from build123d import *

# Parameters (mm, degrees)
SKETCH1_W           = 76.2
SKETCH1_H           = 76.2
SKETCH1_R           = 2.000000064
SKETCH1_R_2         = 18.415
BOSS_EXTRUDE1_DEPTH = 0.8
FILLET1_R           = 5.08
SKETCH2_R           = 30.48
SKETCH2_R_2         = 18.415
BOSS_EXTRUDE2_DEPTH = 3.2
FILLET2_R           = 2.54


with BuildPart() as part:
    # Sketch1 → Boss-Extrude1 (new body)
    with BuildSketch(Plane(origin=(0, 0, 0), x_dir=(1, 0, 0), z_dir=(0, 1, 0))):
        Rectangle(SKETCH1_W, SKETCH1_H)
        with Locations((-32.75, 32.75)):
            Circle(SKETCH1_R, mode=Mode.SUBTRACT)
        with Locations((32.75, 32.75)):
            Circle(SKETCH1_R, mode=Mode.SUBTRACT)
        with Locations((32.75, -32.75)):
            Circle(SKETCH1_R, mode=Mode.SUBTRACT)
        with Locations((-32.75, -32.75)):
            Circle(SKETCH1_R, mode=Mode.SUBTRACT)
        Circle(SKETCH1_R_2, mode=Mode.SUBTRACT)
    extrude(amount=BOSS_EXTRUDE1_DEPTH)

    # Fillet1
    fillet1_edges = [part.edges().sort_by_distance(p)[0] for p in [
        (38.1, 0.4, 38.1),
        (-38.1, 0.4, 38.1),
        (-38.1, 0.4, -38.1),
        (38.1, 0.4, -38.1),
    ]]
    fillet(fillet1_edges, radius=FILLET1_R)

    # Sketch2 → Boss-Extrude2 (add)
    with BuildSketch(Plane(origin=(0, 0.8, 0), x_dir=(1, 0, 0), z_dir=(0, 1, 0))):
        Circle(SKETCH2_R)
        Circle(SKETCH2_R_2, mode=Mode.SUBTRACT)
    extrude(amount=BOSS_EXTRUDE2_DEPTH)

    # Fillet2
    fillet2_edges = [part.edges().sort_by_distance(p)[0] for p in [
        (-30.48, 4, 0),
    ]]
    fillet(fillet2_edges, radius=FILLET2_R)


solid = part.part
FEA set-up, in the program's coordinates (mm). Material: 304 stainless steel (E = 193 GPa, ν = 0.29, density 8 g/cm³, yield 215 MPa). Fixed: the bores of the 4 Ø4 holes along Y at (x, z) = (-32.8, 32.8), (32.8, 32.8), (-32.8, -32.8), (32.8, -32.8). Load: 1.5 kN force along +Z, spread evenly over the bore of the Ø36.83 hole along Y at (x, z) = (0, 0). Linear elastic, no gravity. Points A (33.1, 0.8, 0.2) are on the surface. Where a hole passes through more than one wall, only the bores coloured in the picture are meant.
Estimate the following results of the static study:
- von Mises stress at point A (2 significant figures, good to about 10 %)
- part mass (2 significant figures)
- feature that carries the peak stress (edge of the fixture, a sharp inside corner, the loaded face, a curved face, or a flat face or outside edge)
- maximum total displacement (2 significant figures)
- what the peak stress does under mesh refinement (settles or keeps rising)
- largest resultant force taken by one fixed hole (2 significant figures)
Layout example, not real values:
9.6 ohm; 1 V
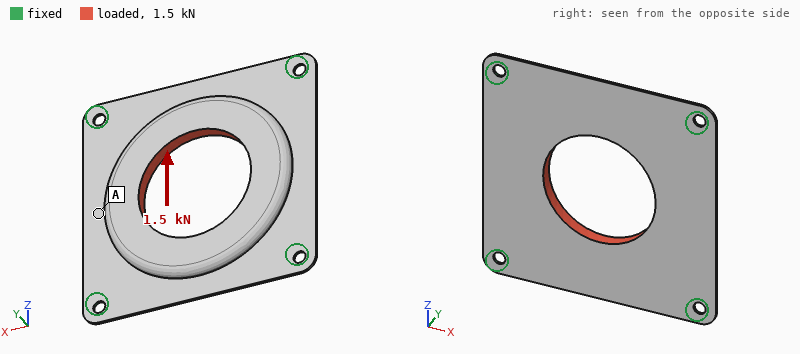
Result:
13 MPa; 75 g; edge of the fixture; 48 µm; keeps rising; 400 N
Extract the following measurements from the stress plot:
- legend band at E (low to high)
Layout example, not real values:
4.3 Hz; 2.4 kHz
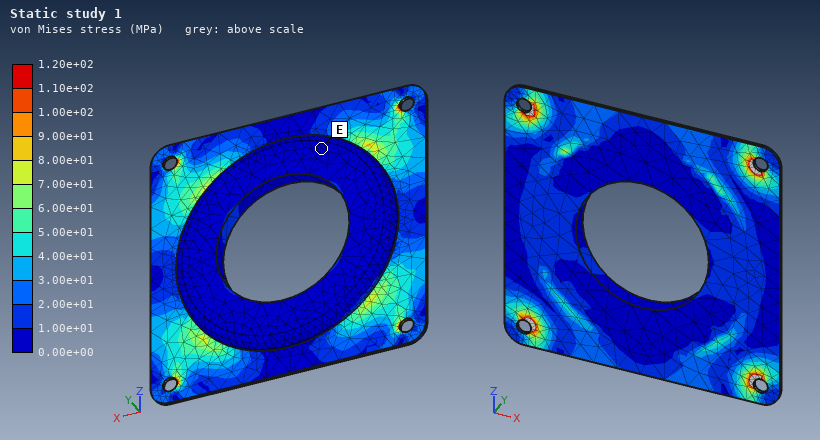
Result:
0.00e+00 to 1.00e+01 MPa
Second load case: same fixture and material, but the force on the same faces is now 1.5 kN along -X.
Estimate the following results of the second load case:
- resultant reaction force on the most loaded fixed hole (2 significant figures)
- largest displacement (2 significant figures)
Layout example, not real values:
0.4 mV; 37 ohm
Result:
400 N; 49 µm
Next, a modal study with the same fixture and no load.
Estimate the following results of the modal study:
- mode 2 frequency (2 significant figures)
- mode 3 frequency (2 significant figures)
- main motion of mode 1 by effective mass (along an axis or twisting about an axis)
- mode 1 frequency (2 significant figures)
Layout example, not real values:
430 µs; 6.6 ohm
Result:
1300 Hz; 1300 Hz; along Y; 880 Hz
